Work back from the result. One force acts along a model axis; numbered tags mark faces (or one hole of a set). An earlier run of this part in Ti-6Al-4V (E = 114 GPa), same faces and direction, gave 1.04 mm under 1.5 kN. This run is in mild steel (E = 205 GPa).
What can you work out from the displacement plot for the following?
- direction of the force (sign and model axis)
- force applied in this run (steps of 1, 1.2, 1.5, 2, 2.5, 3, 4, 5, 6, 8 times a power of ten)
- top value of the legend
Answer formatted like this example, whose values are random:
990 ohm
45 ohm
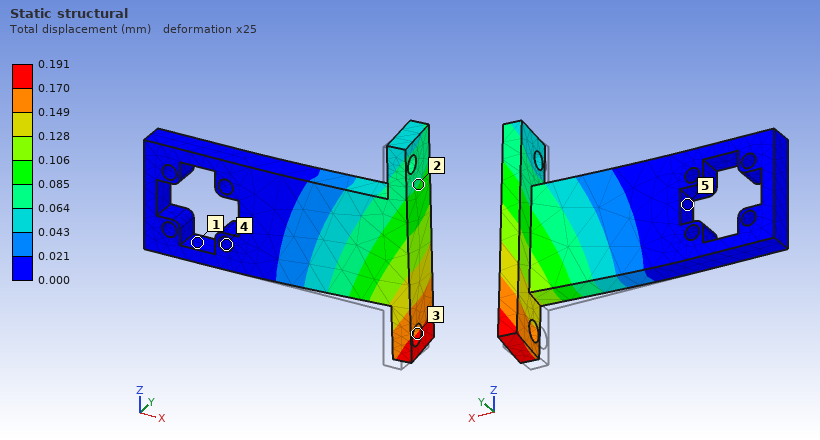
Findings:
+Y
500 N
0.191 mm
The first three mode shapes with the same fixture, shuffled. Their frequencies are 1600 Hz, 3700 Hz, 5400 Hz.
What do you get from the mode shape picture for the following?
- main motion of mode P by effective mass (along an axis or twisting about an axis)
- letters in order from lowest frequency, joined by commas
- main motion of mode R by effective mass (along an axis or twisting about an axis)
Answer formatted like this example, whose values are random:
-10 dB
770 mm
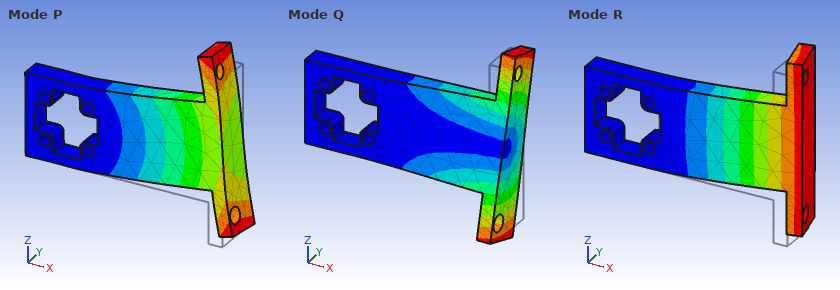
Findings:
along Z
R, Q, P
along Y
